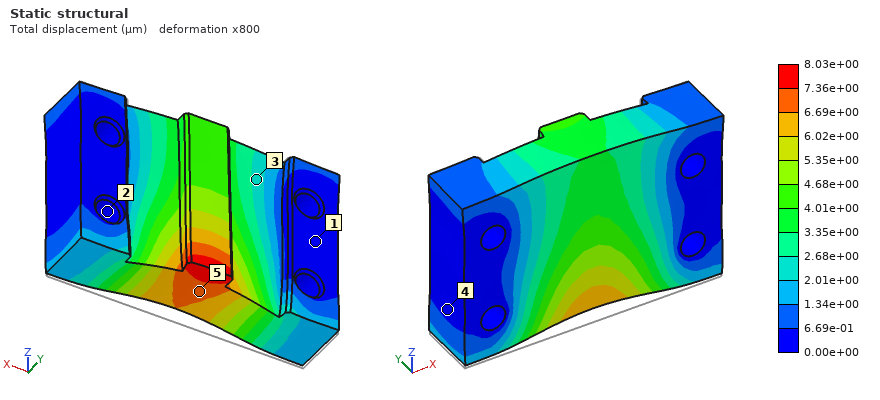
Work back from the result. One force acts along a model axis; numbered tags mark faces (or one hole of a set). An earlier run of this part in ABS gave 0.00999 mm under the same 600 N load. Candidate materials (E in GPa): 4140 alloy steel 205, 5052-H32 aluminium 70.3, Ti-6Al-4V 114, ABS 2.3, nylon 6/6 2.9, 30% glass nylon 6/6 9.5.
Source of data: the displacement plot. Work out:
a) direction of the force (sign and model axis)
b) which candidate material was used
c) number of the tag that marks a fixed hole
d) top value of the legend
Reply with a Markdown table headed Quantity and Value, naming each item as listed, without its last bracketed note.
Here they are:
| Quantity | Value |
|---|---|
| direction of the force | +Z |
| which candidate material was used | nylon 6/6 |
| number of the tag that marks a fixed hole | 2 |
| top value of the legend | 8.03e+00 µm |
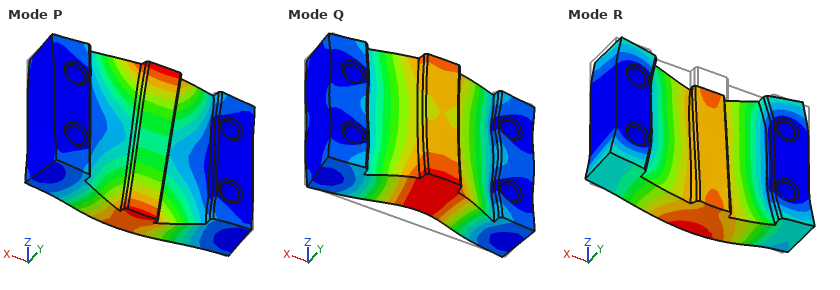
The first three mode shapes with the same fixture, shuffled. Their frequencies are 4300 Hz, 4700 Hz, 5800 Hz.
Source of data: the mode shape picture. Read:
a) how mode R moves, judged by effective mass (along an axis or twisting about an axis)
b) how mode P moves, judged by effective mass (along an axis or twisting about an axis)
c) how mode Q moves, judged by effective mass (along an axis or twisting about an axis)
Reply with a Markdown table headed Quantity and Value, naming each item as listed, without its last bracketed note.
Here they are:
| Quantity | Value |
|---|---|
| how mode R moves, judged by effective mass | along Z |
| how mode P moves, judged by effective mass | twisting about X |
| how mode Q moves, judged by effective mass | along Y |
